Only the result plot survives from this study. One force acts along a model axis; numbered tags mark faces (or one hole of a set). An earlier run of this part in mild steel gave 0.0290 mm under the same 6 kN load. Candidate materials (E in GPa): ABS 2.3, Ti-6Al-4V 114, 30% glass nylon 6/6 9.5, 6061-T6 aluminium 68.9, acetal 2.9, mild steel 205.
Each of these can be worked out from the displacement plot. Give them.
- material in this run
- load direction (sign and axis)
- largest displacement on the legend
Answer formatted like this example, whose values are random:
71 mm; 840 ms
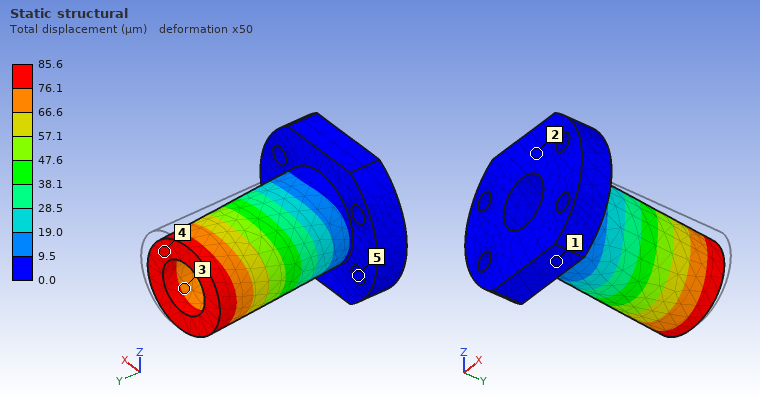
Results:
6061-T6 aluminium; -X; 85.6 µm
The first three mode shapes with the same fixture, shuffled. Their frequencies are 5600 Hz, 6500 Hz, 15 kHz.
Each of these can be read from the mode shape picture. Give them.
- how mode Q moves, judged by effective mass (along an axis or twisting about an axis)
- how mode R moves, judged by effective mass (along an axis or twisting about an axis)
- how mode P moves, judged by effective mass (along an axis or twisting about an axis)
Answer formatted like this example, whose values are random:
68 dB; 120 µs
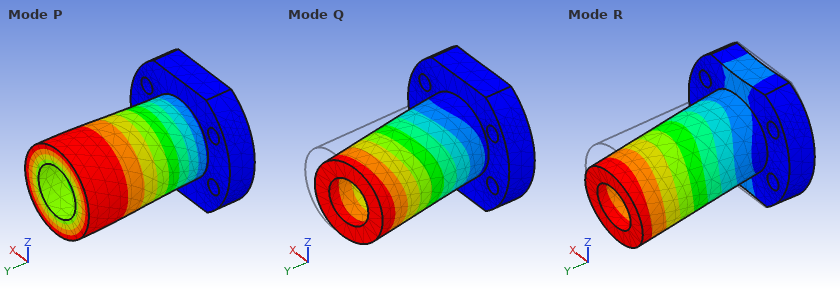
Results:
along X; along Z; twisting about Y
